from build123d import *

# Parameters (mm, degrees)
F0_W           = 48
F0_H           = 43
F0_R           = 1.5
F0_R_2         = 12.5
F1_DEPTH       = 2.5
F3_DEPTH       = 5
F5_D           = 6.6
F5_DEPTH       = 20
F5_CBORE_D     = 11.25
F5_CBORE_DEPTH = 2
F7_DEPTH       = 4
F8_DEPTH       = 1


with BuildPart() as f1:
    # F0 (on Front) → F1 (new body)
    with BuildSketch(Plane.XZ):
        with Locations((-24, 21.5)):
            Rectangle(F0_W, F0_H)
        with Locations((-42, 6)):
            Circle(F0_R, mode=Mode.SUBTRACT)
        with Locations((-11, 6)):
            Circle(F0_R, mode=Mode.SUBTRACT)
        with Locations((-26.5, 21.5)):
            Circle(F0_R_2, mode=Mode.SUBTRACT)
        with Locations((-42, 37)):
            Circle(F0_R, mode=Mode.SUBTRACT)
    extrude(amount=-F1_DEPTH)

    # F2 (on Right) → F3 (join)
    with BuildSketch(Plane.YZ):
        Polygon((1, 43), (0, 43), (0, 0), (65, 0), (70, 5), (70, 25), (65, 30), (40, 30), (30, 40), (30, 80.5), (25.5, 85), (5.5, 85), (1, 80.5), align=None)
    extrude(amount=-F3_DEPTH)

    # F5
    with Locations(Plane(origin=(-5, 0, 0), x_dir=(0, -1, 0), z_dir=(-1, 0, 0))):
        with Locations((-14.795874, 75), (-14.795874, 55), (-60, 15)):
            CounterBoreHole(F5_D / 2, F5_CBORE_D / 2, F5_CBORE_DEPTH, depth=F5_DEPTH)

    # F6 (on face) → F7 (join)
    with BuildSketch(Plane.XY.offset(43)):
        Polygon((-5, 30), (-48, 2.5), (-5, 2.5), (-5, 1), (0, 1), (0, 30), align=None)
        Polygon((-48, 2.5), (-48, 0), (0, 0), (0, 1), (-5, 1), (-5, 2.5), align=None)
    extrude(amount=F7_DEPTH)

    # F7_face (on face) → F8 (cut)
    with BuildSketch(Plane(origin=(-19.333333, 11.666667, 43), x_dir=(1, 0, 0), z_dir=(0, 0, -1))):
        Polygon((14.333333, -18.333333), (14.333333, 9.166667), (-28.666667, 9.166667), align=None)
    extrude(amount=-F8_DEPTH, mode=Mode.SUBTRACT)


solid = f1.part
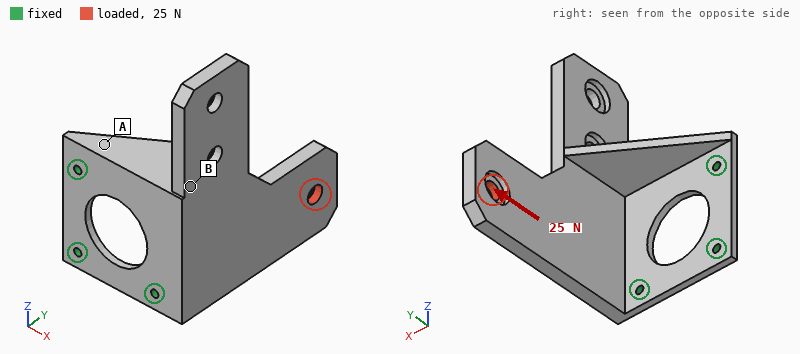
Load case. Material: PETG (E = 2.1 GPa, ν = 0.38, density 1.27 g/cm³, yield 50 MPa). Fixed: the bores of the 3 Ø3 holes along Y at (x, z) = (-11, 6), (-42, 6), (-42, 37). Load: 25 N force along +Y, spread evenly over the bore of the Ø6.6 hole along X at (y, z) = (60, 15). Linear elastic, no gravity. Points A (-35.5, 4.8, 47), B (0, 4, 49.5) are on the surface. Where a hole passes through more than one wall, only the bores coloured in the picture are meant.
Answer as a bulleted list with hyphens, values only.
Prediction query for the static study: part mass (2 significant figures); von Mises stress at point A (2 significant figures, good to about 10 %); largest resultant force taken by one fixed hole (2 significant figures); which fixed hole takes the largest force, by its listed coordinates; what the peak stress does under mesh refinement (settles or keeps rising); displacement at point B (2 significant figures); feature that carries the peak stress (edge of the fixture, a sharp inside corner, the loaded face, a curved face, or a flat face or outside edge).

- 29 g
- 1.5 MPa
- 24 N
- (-11, 6)
- keeps rising
- 0.60 mm
- edge of the fixture
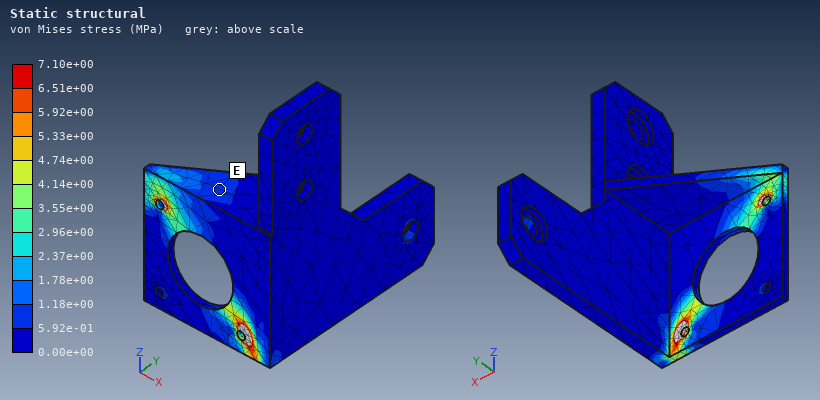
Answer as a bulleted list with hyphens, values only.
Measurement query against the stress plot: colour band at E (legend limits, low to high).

- 5.92e-01 to 1.18e+00 MPa
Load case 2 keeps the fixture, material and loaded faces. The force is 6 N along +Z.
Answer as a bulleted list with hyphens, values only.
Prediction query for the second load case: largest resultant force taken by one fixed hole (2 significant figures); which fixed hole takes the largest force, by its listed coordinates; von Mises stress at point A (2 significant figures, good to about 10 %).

- 7.8 N
- (-11, 6)
- 1.6 MPa
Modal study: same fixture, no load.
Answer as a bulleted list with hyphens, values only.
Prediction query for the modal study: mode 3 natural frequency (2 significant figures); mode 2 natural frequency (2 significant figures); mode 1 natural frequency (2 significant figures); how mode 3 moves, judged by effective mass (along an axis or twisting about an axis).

- 530 Hz
- 260 Hz
- 95 Hz
- along X
